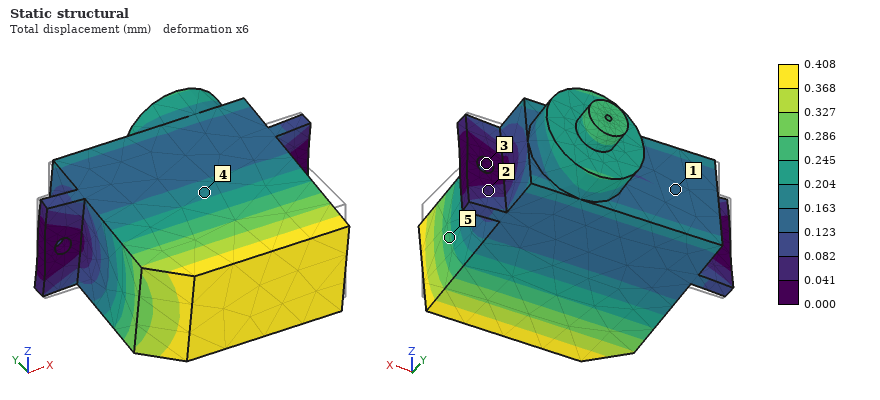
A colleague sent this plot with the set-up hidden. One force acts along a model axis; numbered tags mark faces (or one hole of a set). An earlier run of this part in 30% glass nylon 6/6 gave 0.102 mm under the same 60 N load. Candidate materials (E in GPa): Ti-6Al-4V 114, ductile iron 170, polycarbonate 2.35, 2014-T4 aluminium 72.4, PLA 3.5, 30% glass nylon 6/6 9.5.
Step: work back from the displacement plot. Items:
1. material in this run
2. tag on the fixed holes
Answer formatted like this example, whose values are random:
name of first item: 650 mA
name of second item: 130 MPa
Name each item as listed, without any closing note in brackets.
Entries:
material in this run: polycarbonate
tag on the fixed holes: 3
